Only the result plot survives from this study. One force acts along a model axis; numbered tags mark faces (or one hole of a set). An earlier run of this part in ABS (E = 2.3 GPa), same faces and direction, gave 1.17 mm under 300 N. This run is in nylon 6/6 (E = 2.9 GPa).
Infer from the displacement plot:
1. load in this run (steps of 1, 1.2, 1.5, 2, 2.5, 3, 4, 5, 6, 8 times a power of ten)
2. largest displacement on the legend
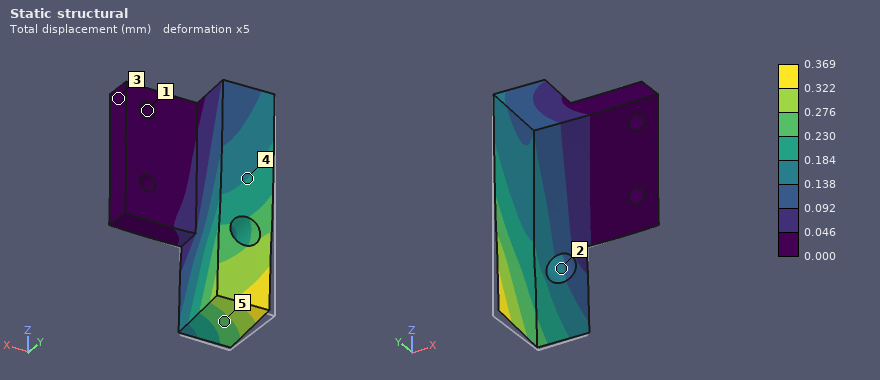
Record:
120 N
0.369 mm
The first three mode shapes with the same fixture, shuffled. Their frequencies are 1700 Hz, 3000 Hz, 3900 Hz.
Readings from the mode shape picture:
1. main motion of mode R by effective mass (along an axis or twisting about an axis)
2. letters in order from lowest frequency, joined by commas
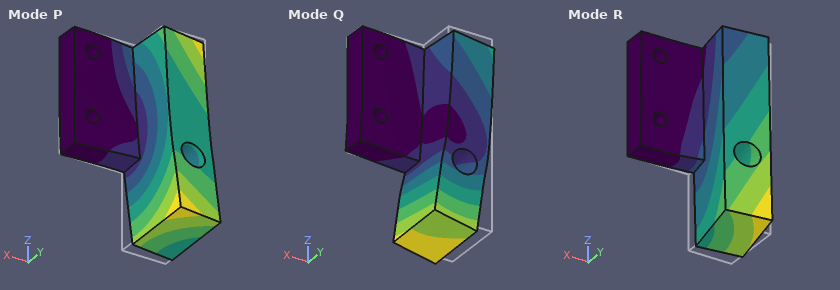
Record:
along Y
R, P, Q
